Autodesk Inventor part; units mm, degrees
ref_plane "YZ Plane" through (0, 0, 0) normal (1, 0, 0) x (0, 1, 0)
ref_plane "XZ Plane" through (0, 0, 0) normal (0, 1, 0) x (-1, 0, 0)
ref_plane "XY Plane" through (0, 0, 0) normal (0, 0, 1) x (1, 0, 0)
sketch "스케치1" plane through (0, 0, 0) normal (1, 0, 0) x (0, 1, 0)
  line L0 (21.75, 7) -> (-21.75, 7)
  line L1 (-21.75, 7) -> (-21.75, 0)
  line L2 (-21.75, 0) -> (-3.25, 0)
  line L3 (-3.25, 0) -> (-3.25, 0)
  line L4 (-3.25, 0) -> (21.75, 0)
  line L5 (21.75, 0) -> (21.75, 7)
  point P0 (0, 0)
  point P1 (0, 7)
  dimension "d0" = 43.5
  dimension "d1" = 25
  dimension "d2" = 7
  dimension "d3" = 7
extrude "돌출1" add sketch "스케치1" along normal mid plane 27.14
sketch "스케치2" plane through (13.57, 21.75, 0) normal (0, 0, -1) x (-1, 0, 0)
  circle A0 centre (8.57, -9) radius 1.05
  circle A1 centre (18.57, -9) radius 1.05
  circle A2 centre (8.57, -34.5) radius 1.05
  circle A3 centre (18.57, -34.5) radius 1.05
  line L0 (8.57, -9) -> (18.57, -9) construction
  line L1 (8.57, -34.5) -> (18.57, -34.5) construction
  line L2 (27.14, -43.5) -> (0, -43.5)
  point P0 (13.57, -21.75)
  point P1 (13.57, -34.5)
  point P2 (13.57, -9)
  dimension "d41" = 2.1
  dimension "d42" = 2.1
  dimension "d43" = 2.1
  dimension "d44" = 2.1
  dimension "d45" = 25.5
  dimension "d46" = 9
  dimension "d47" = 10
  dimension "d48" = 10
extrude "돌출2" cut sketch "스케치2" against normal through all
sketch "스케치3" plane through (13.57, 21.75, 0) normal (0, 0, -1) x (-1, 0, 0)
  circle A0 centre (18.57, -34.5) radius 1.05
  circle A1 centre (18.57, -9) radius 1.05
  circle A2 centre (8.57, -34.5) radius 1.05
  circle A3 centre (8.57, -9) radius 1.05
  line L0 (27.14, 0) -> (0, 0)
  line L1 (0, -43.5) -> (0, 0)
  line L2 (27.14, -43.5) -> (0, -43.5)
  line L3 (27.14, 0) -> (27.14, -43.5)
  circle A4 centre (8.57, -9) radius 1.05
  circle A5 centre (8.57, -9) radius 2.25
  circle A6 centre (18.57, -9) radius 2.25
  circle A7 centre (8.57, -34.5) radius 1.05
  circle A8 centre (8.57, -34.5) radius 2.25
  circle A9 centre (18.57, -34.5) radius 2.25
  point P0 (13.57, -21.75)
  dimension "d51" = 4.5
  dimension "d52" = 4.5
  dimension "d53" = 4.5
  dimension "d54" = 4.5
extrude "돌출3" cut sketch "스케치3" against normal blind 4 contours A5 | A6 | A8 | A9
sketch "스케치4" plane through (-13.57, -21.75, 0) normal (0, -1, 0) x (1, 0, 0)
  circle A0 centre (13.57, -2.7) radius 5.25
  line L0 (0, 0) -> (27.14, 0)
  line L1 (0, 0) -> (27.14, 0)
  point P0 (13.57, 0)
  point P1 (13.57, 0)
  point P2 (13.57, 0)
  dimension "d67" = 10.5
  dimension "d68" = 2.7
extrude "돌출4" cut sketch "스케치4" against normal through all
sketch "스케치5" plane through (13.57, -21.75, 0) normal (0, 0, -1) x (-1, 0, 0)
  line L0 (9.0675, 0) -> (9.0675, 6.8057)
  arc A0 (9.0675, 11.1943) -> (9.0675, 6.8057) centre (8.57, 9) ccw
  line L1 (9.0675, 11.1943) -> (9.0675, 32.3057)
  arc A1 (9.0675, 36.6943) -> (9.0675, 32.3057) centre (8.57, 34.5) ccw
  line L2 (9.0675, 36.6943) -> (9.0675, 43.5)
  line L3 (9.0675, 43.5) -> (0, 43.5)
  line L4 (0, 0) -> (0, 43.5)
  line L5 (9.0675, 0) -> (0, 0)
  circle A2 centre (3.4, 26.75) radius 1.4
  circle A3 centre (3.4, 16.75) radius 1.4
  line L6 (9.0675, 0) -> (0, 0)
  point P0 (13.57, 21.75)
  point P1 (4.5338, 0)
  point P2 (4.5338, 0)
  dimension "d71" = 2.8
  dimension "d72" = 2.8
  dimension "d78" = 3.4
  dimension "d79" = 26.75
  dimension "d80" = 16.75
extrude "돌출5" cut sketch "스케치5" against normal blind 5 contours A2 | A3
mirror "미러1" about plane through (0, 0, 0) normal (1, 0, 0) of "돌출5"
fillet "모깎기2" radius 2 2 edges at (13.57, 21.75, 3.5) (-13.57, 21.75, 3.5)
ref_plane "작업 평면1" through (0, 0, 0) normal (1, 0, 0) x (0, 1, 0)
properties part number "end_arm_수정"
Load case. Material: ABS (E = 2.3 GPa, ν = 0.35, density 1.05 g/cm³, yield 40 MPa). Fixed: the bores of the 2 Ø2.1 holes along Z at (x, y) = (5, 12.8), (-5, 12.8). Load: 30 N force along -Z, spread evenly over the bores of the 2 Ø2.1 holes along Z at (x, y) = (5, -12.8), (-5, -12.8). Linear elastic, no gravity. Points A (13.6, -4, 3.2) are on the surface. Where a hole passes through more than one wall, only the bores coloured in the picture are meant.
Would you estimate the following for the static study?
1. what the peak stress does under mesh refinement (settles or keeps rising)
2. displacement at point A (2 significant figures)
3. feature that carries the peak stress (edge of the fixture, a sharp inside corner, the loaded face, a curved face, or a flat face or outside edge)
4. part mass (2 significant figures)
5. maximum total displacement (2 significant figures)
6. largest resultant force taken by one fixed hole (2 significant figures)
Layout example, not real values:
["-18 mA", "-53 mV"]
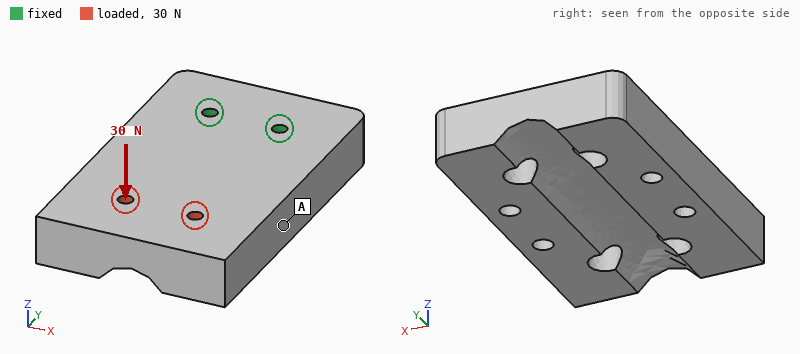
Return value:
["keeps rising", "0.23 mm", "edge of the fixture", "7.5 g", "0.55 mm", "15 N"]
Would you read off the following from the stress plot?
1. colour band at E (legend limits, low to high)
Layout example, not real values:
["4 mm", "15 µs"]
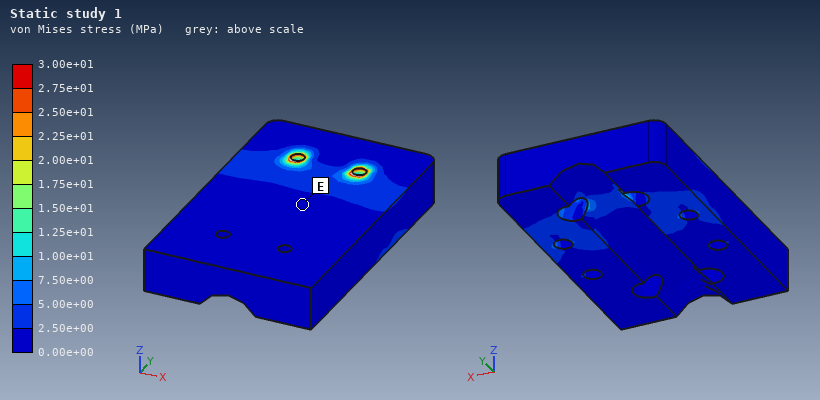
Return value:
["0.00e+00 to 2.50e+00 MPa"]
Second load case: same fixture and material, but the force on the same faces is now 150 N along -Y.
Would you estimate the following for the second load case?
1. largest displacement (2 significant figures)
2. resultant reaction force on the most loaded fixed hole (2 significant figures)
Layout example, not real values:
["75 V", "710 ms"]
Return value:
["90 µm", "76 N"]
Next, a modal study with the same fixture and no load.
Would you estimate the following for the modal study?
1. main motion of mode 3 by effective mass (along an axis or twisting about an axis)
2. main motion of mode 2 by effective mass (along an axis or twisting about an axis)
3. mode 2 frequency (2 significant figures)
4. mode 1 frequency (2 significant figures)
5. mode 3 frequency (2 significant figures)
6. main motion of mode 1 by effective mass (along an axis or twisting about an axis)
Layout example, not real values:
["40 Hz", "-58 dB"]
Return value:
["twisting about Y", "along X", "2200 Hz", "730 Hz", "2400 Hz", "along Z"]
